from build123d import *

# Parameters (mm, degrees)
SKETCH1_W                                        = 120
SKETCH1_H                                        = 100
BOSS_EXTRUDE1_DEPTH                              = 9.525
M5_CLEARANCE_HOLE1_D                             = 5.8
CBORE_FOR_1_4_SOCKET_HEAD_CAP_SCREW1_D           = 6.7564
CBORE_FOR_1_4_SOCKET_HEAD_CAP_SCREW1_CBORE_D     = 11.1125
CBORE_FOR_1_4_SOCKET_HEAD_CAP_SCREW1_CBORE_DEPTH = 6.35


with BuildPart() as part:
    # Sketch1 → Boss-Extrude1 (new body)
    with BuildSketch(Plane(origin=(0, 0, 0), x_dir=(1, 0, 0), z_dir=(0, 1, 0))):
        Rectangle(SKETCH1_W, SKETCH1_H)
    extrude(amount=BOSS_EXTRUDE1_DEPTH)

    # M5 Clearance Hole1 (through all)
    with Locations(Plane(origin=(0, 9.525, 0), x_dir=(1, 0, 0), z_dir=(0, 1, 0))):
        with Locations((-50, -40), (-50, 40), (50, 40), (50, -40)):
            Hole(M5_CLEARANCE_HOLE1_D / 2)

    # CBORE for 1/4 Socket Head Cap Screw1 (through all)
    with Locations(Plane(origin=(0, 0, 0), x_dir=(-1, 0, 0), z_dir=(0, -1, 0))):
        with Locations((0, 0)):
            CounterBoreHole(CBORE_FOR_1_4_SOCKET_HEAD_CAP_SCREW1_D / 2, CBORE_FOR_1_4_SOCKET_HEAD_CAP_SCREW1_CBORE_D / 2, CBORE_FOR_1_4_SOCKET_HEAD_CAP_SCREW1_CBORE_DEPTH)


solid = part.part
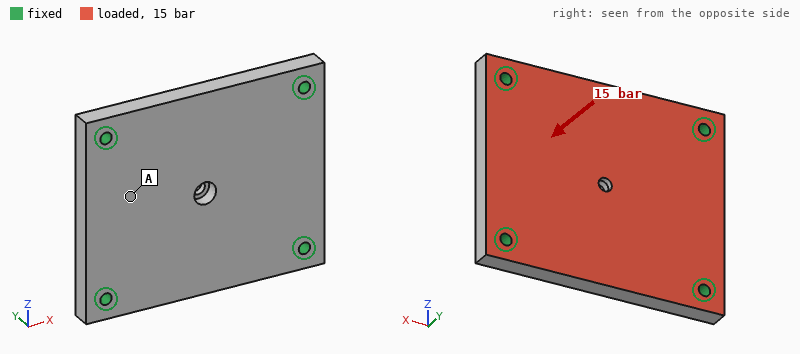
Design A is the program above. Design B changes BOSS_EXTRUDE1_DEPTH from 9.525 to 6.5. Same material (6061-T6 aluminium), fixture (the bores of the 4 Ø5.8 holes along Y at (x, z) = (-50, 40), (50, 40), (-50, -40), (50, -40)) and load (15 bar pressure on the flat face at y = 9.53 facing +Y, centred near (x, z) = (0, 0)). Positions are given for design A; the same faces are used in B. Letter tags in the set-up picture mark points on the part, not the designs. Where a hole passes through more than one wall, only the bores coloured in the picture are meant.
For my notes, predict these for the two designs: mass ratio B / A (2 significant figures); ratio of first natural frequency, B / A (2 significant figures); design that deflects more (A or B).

0.68
0.72
B
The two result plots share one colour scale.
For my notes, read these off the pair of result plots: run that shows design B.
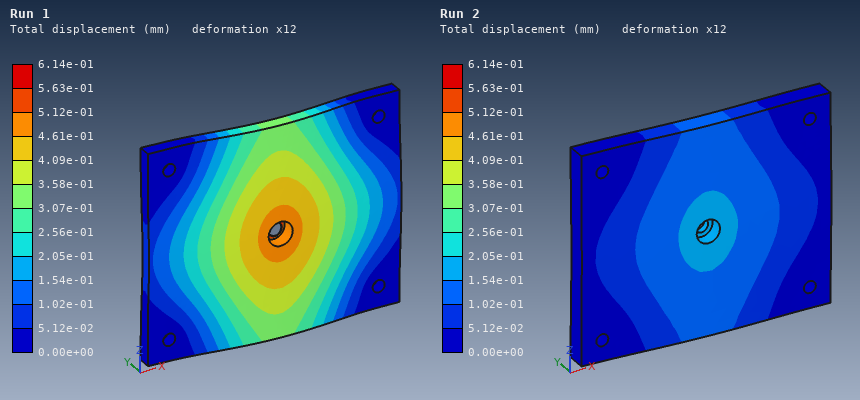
Run 1
